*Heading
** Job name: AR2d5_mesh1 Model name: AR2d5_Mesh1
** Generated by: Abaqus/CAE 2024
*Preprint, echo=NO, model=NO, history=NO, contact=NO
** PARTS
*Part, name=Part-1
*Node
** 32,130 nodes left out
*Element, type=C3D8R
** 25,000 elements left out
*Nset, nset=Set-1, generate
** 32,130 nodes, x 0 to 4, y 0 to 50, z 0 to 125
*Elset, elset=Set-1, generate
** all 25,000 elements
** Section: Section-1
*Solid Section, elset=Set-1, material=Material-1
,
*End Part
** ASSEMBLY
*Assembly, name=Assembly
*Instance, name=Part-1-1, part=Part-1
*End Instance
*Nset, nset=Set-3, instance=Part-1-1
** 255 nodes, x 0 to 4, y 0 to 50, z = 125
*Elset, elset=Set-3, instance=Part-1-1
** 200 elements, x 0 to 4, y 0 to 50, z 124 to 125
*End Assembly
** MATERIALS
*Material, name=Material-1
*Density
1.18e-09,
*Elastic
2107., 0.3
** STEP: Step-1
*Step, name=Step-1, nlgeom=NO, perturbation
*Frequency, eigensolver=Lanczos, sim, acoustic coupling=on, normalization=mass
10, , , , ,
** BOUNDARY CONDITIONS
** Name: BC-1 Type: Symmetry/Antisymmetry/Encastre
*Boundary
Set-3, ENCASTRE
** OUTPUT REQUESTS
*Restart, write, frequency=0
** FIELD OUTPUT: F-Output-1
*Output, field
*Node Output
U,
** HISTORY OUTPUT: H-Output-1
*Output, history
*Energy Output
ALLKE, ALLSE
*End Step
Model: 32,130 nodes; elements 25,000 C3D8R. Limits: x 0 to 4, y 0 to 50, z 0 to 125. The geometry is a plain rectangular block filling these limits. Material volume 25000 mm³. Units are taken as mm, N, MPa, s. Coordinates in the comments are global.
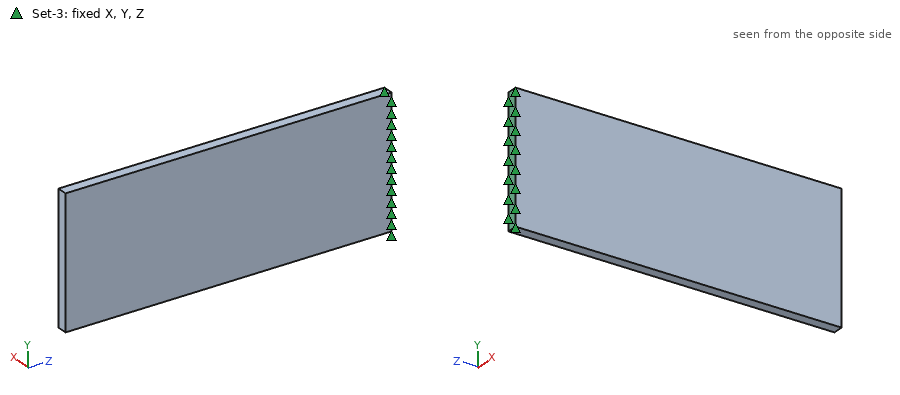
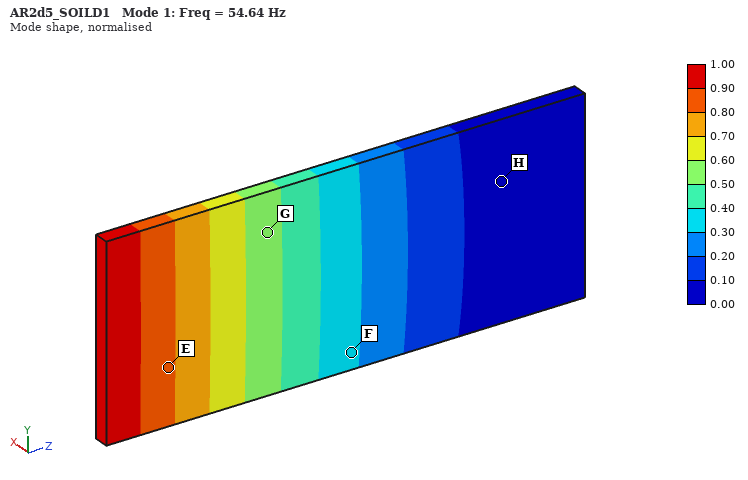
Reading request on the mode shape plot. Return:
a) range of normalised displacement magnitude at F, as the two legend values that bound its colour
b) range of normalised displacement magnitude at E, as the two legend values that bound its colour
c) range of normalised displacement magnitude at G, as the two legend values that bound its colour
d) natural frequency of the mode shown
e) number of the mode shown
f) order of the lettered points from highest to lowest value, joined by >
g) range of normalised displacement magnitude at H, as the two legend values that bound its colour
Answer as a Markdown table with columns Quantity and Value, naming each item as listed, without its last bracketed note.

| Quantity | Value |
|---|---|
| range of normalised displacement magnitude at F, as the two legend values that bound its colour | 0.30 to 0.40 |
| range of normalised displacement magnitude at E, as the two legend values that bound its colour | 0.80 to 0.90 |
| range of normalised displacement magnitude at G, as the two legend values that bound its colour | 0.50 to 0.60 |
| natural frequency of the mode shown | 54.64 Hz |
| number of the mode shown | 1 |
| order of the lettered points from highest to lowest value, joined by > | E > G > F > H |
| range of normalised displacement magnitude at H, as the two legend values that bound its colour | 0.00 to 0.10 |
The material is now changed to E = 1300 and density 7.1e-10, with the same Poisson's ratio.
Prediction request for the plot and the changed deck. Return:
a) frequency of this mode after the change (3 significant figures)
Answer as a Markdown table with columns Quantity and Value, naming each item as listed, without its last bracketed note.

| Quantity | Value |
|---|---|
| frequency of this mode after the change | 55.3 Hz |
